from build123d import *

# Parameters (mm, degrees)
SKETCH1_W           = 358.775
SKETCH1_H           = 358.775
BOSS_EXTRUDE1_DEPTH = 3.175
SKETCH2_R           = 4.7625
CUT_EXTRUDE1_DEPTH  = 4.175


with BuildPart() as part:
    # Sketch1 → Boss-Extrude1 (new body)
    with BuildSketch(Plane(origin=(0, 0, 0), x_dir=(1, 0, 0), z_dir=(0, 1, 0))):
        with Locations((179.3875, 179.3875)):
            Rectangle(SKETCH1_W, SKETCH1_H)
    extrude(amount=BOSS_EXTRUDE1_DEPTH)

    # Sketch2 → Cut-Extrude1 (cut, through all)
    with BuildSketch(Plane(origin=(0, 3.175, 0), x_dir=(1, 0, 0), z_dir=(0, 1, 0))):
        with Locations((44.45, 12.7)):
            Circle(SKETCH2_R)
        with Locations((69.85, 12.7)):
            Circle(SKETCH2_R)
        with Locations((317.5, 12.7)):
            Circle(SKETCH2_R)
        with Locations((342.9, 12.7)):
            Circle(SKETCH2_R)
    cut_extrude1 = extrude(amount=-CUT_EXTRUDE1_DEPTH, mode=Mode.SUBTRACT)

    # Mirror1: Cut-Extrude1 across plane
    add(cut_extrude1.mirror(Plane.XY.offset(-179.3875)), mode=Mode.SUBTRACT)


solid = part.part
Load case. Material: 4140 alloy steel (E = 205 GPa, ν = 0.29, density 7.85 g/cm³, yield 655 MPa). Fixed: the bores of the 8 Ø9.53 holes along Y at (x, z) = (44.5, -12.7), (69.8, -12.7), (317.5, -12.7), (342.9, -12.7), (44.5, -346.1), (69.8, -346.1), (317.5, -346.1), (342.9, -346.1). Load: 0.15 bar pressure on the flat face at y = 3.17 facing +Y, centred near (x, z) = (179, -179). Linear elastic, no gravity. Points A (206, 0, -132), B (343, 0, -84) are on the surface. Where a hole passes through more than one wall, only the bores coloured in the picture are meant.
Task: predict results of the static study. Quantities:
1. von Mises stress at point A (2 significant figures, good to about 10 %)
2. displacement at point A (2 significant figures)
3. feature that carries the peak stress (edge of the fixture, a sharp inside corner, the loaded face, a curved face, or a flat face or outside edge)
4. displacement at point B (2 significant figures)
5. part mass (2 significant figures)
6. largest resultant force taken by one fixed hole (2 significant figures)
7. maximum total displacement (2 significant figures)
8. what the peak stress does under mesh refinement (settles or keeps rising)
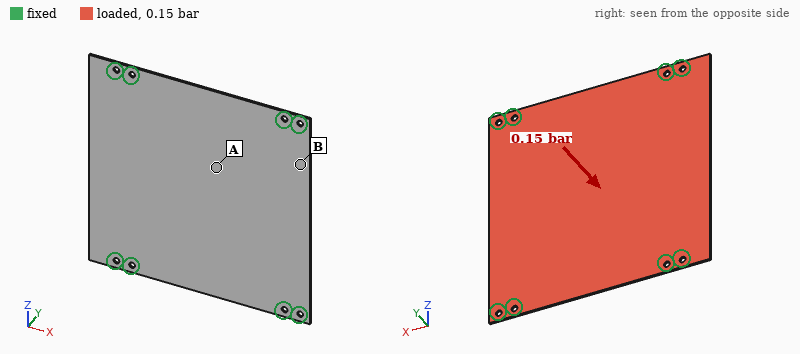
38 MPa
1.4 mm
edge of the fixture
0.50 mm
3.2 kg
490 N
1.5 mm
keeps rising
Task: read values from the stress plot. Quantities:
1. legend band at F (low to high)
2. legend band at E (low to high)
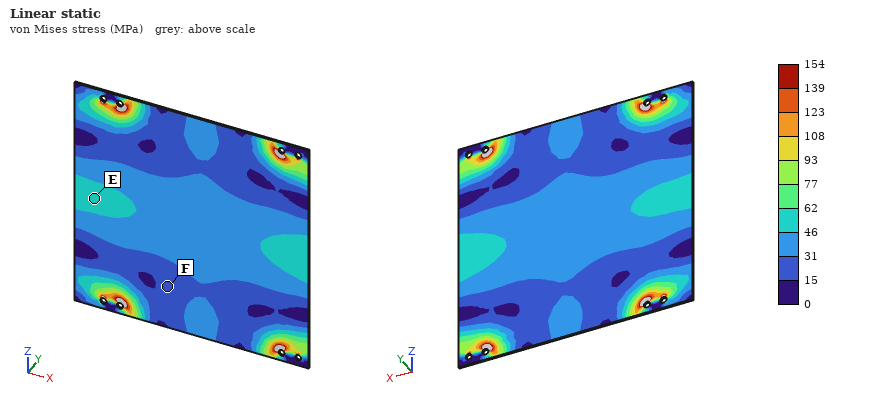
15 to 31 MPa
46 to 62 MPa
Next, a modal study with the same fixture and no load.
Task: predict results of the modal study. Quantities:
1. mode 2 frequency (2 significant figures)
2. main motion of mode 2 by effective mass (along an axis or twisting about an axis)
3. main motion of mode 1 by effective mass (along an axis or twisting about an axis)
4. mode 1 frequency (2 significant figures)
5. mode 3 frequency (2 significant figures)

170 Hz
twisting about Z
along Y
120 Hz
230 Hz
